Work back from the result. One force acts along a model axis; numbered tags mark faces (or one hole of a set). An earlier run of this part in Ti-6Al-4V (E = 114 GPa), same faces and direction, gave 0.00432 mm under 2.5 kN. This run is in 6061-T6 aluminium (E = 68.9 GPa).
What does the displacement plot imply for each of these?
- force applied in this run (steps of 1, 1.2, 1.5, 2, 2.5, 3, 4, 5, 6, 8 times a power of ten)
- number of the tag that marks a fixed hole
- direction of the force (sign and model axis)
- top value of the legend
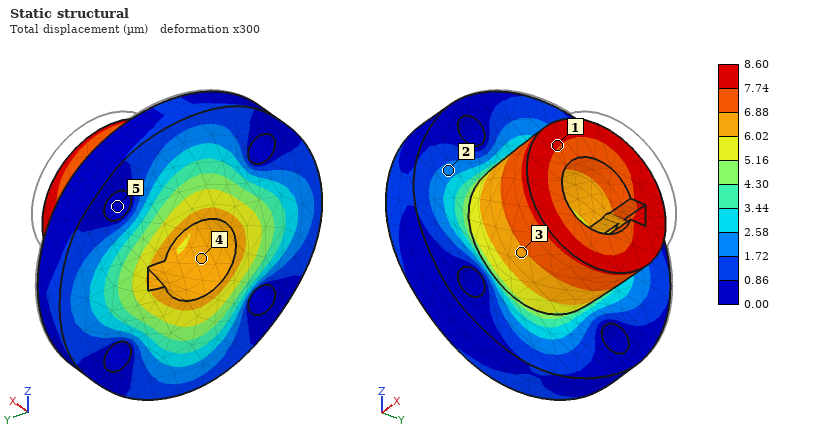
3 kN
5
-X
8.60 µm
